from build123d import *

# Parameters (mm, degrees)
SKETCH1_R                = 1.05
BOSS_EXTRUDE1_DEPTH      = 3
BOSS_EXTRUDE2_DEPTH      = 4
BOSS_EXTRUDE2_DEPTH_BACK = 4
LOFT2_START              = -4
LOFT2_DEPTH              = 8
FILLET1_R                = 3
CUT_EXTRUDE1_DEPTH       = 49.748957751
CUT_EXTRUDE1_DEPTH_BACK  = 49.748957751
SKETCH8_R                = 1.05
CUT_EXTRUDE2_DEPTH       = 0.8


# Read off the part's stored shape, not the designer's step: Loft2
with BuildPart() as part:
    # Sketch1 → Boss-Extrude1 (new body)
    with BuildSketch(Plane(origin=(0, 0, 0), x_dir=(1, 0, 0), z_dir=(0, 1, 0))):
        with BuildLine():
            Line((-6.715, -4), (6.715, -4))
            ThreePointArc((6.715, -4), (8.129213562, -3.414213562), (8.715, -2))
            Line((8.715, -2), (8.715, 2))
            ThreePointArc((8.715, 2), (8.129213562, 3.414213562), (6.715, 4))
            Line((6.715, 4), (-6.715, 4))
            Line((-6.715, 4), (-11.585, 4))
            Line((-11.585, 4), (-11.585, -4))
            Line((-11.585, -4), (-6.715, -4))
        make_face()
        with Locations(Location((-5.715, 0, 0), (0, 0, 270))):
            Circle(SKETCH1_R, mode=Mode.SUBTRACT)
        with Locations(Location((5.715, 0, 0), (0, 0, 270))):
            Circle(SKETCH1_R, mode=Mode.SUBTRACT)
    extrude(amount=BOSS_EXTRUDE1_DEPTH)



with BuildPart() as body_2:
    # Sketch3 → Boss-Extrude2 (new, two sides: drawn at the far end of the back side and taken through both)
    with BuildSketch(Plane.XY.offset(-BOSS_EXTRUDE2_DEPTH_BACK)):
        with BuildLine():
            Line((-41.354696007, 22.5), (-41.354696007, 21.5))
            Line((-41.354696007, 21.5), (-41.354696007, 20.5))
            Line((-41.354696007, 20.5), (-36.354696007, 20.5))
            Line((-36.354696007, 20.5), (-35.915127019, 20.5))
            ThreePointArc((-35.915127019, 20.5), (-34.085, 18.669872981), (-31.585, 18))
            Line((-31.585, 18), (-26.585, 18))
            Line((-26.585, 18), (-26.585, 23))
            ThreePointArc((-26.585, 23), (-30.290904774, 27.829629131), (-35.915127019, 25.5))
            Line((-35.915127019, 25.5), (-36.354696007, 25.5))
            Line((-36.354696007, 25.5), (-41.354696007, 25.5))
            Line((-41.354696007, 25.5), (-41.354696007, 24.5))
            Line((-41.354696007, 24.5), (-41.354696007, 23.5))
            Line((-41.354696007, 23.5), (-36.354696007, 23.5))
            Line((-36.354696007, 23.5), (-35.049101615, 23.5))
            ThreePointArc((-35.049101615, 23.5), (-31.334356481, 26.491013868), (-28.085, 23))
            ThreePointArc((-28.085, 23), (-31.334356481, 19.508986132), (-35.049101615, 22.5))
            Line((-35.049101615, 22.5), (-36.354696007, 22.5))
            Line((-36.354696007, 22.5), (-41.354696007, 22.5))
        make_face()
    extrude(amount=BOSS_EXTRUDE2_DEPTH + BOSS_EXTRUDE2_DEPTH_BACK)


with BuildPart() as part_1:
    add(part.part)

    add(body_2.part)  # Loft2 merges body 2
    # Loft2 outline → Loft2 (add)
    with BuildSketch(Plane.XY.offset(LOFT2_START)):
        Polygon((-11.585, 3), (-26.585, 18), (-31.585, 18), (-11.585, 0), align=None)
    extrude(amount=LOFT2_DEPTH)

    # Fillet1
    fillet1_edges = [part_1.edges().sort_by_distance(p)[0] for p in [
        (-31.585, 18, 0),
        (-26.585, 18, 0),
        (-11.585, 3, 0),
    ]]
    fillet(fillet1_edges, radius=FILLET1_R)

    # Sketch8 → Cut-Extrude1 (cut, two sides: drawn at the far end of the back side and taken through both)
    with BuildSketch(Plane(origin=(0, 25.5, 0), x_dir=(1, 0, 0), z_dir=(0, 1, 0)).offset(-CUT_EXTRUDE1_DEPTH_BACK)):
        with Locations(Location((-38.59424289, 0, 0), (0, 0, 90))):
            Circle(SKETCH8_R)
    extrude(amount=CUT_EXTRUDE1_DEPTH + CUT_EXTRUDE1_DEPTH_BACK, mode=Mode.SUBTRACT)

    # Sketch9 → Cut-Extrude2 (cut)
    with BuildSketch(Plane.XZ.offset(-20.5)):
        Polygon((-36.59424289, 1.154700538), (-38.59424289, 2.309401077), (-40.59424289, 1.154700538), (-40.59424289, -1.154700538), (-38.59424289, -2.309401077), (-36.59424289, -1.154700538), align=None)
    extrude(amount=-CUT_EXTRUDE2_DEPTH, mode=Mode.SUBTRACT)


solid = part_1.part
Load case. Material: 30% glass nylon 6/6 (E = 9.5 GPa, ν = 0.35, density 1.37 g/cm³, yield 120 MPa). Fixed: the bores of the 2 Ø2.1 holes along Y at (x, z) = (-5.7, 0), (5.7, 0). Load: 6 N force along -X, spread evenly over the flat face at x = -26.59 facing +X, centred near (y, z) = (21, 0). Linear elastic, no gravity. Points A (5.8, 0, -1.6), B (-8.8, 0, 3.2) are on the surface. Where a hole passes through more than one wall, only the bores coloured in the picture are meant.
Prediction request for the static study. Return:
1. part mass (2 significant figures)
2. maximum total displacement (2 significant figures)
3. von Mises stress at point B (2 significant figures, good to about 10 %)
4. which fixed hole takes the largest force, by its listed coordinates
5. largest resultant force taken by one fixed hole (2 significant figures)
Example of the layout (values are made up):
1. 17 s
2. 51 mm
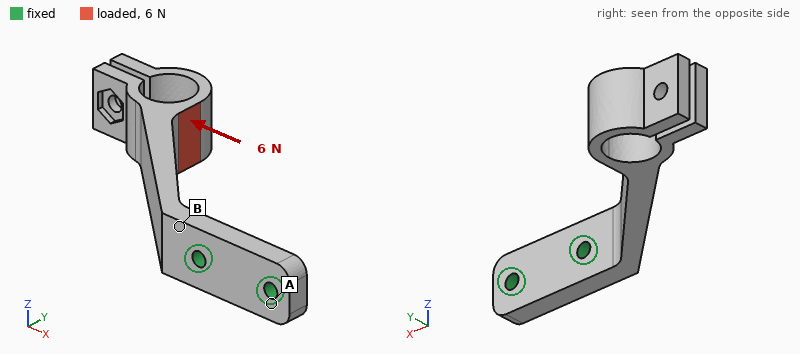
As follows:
1. 2.0 g
2. 0.59 mm
3. 8.9 MPa
4. (-5.7, 0)
5. 5.8 N
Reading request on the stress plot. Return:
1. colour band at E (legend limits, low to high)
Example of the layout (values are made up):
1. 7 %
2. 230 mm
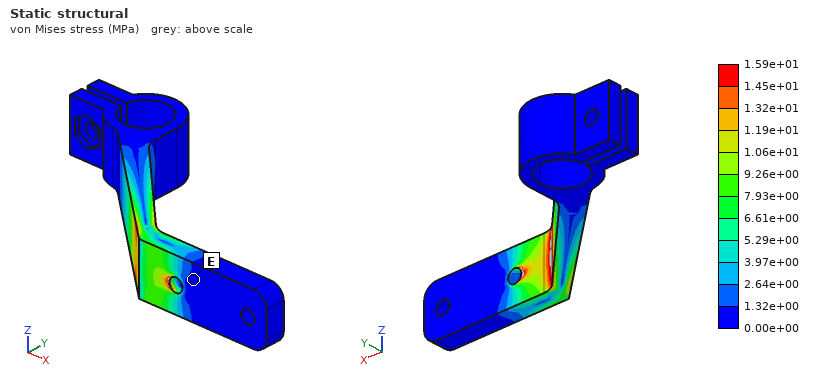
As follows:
1. 0.00e+00 to 1.32e+00 MPa
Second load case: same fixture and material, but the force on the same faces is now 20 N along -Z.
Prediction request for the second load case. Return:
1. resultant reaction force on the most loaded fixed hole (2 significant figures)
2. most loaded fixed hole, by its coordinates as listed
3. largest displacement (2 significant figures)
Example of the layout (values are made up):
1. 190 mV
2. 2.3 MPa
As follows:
1. 42 N
2. (-5.7, 0)
3. 0.56 mm
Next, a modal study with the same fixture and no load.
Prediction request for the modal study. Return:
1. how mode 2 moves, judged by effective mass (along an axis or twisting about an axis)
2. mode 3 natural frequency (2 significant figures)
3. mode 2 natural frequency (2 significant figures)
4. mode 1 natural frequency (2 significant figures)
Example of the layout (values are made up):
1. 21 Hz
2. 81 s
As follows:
1. along Z
2. 2200 Hz
3. 1100 Hz
4. 500 Hz
